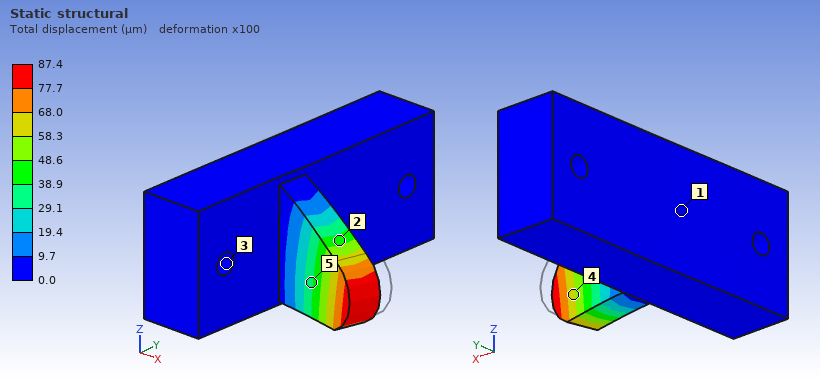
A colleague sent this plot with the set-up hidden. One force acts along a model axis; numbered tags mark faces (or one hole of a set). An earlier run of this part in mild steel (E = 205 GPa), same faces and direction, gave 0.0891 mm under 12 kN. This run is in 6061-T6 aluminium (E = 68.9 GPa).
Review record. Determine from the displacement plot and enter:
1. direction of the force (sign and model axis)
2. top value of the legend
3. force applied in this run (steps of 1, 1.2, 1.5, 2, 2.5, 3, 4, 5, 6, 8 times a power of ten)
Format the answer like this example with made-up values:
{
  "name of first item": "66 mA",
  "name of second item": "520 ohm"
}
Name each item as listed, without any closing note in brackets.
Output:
{
  "direction of the force": "-Y",
  "top value of the legend": "87.4 µm",
  "force applied in this run": "4 kN"
}
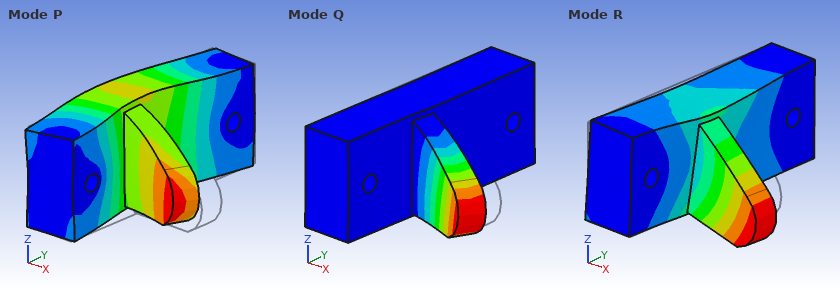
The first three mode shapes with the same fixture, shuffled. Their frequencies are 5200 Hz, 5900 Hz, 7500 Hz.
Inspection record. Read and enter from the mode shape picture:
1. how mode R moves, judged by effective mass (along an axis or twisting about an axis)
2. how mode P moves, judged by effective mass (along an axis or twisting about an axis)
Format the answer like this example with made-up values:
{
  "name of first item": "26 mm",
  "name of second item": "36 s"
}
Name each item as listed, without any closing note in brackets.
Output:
{
  "how mode R moves, judged by effective mass": "along Z",
  "how mode P moves, judged by effective mass": "along X"
}
